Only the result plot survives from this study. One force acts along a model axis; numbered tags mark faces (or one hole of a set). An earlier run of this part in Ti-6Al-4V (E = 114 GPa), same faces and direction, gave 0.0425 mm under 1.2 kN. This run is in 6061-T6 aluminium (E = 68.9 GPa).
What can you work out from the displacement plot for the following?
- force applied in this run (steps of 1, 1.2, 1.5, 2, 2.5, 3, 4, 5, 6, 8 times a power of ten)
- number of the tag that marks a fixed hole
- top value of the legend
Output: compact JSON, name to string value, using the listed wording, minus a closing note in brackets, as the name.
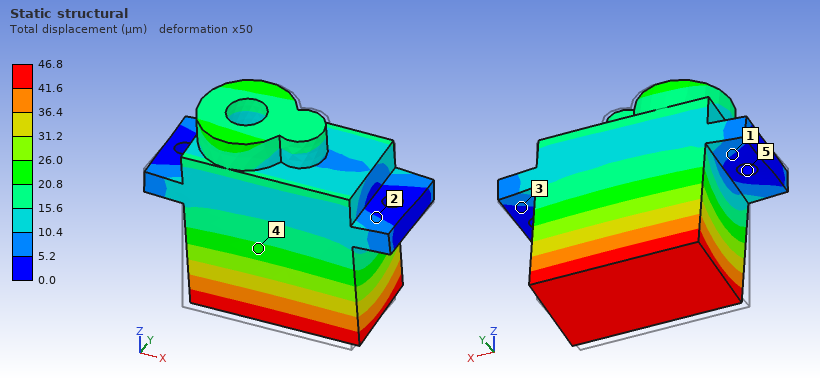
{"force applied in this run": "800 N", "number of the tag that marks a fixed hole": "5", "top value of the legend": "46.8 µm"}
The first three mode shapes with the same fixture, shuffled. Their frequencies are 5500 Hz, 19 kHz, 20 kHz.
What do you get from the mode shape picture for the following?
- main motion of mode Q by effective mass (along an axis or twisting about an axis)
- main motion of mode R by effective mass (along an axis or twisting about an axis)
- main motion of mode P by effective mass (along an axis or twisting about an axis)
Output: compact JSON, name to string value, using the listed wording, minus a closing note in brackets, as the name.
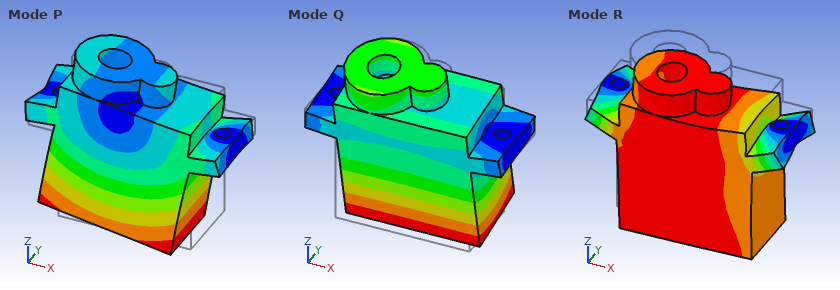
{"main motion of mode Q by effective mass": "along Y", "main motion of mode R by effective mass": "along Z", "main motion of mode P by effective mass": "along X"}
